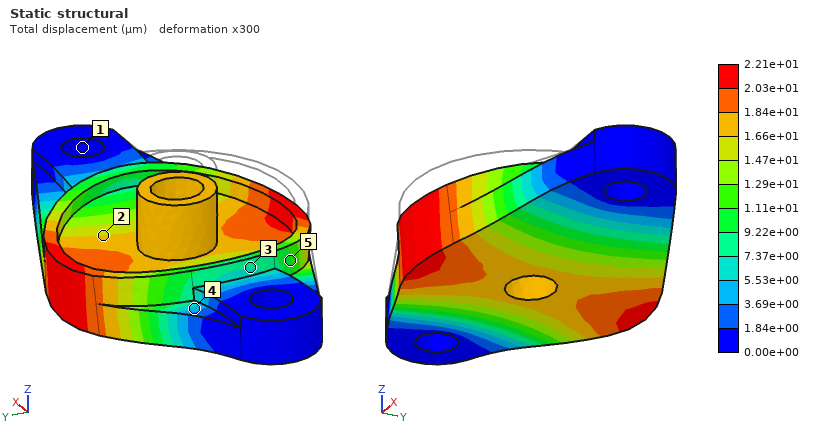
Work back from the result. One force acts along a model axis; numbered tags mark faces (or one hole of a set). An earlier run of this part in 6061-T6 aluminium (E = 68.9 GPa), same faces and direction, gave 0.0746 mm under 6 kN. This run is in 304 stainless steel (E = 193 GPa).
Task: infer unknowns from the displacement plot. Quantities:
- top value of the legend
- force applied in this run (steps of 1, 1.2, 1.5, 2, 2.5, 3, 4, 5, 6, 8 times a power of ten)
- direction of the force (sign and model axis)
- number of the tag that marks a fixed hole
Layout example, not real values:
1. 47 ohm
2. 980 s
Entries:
1. 2.21e+01 µm
2. 5 kN
3. -Z
4. 1
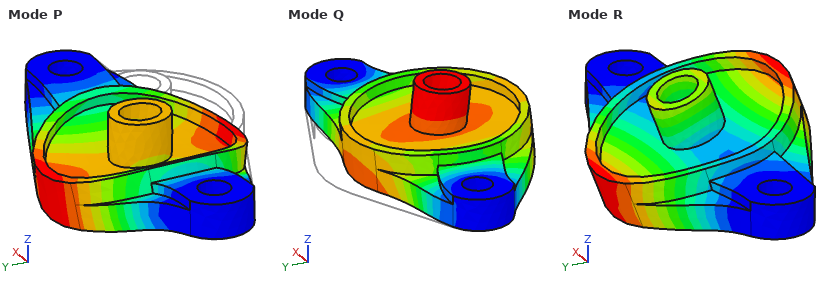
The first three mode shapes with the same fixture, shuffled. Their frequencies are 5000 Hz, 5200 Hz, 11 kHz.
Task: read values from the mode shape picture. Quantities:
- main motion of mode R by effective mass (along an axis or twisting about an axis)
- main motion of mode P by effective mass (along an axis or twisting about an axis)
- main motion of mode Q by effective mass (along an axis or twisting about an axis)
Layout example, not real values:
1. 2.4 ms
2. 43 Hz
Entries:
1. twisting about X
2. along Z
3. along Y
